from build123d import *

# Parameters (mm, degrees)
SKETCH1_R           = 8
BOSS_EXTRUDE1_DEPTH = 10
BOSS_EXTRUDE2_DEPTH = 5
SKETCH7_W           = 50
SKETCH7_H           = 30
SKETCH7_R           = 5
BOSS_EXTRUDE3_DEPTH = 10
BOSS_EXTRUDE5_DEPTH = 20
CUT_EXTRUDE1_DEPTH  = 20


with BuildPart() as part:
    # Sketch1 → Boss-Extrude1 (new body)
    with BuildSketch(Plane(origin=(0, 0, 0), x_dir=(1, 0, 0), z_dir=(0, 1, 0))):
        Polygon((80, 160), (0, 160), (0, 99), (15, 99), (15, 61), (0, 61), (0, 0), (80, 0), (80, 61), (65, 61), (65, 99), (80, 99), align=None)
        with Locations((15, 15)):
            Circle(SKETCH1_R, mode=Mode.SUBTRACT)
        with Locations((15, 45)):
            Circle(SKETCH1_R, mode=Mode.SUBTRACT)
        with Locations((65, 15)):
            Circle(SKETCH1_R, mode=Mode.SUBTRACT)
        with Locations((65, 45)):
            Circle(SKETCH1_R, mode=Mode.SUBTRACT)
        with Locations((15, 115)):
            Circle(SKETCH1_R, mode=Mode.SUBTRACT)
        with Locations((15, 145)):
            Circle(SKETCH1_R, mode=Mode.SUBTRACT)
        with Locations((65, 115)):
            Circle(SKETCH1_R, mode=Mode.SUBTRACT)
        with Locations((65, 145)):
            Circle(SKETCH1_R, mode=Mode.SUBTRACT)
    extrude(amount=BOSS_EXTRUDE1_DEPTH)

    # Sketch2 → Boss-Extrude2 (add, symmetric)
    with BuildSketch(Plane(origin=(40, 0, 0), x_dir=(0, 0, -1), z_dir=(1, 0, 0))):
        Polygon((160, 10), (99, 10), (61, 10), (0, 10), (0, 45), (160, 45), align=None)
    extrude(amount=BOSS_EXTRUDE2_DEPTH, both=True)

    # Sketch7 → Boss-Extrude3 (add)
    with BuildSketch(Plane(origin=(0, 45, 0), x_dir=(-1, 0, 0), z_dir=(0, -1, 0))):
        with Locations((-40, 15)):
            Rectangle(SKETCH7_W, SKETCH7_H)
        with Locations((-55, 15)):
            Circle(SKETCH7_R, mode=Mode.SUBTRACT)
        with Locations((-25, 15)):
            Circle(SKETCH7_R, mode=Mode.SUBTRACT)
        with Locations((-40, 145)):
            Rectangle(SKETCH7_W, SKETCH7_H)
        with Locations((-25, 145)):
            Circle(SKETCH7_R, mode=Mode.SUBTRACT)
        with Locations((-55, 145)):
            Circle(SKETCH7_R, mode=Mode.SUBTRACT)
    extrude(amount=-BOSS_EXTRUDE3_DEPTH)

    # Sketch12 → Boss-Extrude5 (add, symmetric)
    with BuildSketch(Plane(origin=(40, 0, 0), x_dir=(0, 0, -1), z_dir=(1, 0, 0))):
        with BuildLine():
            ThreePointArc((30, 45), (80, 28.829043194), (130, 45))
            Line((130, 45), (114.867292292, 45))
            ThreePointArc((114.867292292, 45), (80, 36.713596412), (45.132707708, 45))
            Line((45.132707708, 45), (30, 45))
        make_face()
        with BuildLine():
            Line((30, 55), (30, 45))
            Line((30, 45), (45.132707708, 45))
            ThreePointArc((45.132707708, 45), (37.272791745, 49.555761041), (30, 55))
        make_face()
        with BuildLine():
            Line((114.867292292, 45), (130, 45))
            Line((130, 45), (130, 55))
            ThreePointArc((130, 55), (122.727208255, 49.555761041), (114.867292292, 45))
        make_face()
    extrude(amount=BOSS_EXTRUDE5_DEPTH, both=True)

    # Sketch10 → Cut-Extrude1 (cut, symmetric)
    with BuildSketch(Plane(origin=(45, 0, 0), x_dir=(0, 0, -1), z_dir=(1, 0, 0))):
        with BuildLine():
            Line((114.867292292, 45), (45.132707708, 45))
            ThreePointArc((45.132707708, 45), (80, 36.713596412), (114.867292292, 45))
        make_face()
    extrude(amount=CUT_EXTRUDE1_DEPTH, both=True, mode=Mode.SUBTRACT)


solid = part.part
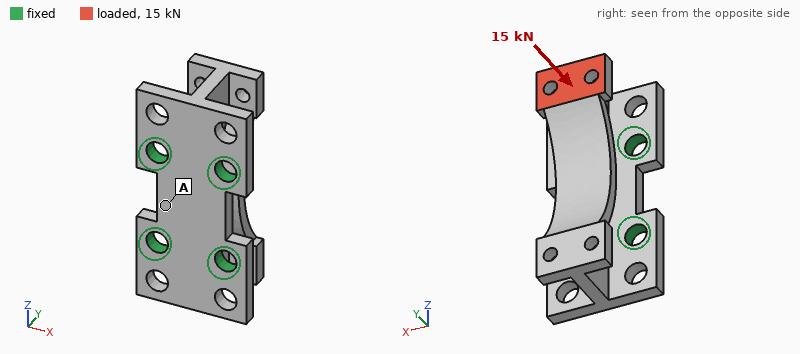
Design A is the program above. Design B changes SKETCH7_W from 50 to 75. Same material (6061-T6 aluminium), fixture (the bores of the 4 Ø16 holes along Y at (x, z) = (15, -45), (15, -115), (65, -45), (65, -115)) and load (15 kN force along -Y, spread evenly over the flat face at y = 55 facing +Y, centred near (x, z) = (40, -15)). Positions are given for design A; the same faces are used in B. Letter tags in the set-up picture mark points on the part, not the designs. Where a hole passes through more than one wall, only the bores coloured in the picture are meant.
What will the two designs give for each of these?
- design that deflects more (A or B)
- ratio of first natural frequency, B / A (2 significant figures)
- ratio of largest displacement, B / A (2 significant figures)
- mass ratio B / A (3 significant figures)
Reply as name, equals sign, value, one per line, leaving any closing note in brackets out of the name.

design that deflects more = B
ratio of first natural frequency, B / A = 0.80
ratio of largest displacement, B / A = 1.7
mass ratio B / A = 1.07
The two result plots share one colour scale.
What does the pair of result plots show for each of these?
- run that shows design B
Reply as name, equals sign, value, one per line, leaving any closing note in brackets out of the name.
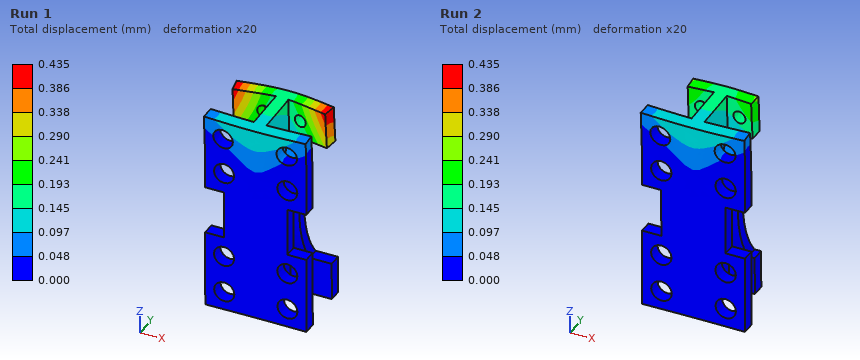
run that shows design B = Run 1
